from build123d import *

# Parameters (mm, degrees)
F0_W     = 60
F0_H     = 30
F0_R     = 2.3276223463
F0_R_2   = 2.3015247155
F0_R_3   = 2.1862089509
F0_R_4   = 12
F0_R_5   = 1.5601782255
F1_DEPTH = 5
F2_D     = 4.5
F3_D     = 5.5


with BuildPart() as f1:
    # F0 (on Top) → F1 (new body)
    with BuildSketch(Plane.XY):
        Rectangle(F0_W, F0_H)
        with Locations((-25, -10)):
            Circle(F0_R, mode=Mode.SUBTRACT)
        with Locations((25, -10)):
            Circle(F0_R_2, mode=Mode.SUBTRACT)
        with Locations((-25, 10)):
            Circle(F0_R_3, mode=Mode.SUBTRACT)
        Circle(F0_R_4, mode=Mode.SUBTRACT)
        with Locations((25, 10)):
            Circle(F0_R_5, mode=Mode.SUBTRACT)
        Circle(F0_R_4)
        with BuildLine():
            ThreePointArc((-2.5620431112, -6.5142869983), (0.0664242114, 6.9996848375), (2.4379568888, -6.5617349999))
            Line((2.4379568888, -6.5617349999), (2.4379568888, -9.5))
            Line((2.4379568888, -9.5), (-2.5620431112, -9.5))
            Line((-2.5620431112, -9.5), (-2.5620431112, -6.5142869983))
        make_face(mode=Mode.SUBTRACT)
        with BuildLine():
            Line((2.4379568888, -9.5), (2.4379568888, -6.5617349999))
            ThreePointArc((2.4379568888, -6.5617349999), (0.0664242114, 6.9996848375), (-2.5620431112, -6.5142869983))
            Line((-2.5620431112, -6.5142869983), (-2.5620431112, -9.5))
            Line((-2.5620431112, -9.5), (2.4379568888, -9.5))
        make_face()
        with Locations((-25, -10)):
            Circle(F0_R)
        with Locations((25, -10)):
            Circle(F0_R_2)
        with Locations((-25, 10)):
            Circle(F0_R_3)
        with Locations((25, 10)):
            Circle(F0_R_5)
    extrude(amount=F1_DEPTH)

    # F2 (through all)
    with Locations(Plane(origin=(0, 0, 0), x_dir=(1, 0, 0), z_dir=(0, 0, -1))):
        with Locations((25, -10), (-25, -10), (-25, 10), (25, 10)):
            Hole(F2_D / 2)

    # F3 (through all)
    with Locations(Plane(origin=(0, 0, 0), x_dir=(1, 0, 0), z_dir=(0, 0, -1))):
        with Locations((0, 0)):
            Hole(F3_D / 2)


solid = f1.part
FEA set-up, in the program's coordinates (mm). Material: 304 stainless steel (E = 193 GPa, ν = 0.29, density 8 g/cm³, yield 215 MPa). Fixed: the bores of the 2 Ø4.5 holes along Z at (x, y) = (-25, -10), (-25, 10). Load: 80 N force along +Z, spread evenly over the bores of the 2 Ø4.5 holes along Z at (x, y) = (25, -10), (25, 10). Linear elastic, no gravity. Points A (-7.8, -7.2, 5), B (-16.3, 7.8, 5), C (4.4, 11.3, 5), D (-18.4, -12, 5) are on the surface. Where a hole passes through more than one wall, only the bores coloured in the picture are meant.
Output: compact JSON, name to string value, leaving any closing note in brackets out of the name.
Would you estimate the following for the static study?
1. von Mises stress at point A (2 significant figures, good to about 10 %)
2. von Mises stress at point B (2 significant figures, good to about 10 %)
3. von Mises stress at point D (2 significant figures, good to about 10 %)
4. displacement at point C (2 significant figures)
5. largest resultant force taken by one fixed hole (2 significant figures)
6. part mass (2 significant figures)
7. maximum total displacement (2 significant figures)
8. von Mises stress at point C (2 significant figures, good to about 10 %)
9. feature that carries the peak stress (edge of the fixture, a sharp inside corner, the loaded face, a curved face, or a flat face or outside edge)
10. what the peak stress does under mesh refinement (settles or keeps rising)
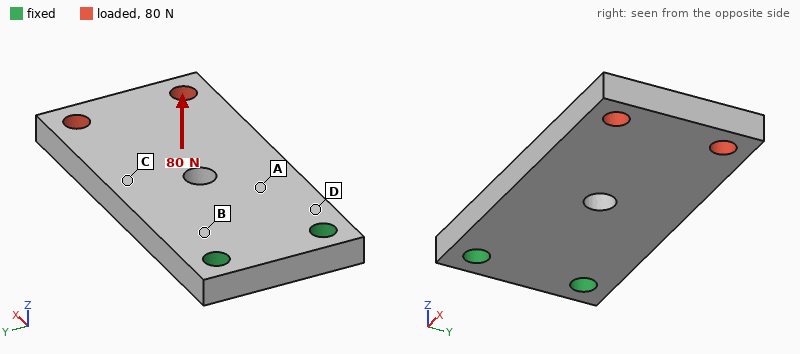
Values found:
{"von Mises stress at point A": "21 MPa", "von Mises stress at point B": "25 MPa", "von Mises stress at point D": "30 MPa", "displacement at point C": "23 µm", "largest resultant force taken by one fixed hole": "40 N", "part mass": "69 g", "maximum total displacement": "64 µm", "von Mises stress at point C": "15 MPa", "feature that carries the peak stress": "edge of the fixture", "what the peak stress does under mesh refinement": "keeps rising"}
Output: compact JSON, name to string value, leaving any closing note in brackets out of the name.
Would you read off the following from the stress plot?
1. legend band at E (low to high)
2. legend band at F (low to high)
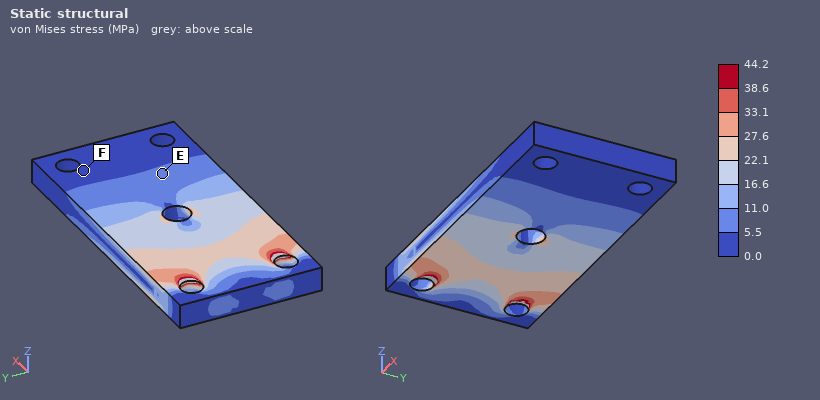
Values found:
{"legend band at E": "5.5 to 11.0 MPa", "legend band at F": "0.0 to 5.5 MPa"}
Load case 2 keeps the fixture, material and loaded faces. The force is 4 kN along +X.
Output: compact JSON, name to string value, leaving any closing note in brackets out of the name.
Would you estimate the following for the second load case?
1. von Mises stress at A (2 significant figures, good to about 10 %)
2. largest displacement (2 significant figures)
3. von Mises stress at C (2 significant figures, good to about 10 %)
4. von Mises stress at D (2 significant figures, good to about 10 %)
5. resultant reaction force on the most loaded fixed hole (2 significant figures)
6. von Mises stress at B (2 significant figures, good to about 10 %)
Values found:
{"von Mises stress at A": "29 MPa", "largest displacement": "9.4 µm", "von Mises stress at C": "29 MPa", "von Mises stress at D": "34 MPa", "resultant reaction force on the most loaded fixed hole": "2.0 kN", "von Mises stress at B": "30 MPa"}
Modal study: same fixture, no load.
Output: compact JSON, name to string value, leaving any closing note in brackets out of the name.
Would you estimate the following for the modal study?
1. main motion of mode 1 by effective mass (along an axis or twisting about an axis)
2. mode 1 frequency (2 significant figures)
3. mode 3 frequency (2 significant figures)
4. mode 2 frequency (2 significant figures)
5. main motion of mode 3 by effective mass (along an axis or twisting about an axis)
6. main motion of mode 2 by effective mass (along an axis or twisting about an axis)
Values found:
{"main motion of mode 1 by effective mass": "along Z", "mode 1 frequency": "1400 Hz", "mode 3 frequency": "6700 Hz", "mode 2 frequency": "5100 Hz", "main motion of mode 3 by effective mass": "along Y", "main motion of mode 2 by effective mass": "twisting about X"}
